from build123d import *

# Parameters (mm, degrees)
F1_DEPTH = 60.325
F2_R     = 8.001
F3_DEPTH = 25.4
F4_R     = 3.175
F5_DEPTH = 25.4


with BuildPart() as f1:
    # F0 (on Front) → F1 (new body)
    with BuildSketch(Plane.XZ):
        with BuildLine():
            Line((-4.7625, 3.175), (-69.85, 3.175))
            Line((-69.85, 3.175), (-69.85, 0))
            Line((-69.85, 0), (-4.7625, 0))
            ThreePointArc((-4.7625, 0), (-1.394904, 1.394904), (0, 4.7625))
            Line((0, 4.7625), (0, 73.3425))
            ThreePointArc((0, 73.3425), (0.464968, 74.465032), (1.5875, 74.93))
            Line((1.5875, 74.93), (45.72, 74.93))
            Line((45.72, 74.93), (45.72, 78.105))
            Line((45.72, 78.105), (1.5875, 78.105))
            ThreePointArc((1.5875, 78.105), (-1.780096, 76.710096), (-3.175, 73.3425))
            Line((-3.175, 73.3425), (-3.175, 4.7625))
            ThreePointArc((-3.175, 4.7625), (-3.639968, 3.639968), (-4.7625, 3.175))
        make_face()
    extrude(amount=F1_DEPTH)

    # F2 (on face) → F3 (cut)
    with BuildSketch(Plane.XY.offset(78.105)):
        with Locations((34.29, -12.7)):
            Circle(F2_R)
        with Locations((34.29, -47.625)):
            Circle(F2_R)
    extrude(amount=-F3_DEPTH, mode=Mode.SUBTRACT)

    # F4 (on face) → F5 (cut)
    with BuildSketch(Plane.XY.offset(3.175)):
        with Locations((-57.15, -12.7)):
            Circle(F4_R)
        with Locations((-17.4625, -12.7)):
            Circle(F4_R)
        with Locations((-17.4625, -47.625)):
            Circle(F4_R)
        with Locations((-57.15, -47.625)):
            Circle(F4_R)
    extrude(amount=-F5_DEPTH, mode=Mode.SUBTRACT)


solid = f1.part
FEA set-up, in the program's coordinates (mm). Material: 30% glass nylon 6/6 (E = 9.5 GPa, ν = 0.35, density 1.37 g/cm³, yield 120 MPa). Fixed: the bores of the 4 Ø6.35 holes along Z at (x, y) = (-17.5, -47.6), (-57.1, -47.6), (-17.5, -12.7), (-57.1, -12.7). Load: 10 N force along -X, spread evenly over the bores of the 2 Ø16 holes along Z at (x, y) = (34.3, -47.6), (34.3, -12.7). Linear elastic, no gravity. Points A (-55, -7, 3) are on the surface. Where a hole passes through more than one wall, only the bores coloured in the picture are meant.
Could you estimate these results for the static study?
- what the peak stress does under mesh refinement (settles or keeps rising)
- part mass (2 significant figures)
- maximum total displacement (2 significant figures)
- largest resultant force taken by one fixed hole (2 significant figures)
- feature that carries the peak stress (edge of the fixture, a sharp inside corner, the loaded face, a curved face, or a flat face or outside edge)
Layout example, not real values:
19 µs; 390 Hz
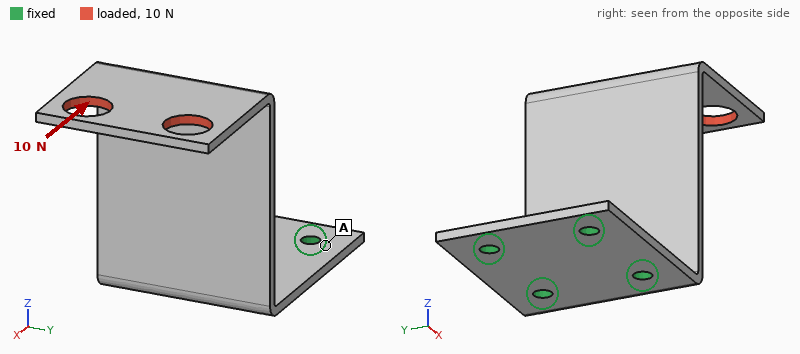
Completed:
keeps rising; 47 g; 1.8 mm; 5.5 N; edge of the fixture
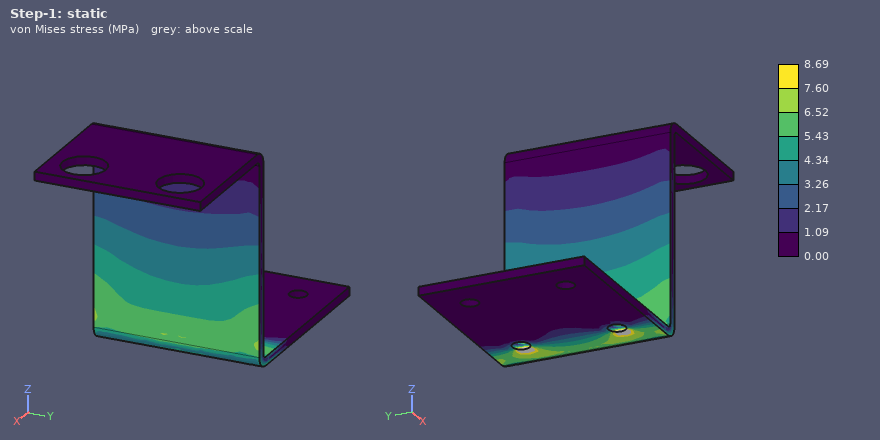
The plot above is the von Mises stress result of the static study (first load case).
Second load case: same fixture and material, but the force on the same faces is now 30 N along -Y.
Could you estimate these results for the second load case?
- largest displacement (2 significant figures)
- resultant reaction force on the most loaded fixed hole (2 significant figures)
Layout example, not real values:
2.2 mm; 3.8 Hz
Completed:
1.5 mm; 68 N
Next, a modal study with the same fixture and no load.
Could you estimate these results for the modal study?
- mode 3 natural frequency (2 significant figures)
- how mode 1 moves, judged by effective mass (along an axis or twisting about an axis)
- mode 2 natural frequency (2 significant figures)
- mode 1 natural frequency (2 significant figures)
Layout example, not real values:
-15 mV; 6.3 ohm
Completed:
440 Hz; along X; 290 Hz; 100 Hz
